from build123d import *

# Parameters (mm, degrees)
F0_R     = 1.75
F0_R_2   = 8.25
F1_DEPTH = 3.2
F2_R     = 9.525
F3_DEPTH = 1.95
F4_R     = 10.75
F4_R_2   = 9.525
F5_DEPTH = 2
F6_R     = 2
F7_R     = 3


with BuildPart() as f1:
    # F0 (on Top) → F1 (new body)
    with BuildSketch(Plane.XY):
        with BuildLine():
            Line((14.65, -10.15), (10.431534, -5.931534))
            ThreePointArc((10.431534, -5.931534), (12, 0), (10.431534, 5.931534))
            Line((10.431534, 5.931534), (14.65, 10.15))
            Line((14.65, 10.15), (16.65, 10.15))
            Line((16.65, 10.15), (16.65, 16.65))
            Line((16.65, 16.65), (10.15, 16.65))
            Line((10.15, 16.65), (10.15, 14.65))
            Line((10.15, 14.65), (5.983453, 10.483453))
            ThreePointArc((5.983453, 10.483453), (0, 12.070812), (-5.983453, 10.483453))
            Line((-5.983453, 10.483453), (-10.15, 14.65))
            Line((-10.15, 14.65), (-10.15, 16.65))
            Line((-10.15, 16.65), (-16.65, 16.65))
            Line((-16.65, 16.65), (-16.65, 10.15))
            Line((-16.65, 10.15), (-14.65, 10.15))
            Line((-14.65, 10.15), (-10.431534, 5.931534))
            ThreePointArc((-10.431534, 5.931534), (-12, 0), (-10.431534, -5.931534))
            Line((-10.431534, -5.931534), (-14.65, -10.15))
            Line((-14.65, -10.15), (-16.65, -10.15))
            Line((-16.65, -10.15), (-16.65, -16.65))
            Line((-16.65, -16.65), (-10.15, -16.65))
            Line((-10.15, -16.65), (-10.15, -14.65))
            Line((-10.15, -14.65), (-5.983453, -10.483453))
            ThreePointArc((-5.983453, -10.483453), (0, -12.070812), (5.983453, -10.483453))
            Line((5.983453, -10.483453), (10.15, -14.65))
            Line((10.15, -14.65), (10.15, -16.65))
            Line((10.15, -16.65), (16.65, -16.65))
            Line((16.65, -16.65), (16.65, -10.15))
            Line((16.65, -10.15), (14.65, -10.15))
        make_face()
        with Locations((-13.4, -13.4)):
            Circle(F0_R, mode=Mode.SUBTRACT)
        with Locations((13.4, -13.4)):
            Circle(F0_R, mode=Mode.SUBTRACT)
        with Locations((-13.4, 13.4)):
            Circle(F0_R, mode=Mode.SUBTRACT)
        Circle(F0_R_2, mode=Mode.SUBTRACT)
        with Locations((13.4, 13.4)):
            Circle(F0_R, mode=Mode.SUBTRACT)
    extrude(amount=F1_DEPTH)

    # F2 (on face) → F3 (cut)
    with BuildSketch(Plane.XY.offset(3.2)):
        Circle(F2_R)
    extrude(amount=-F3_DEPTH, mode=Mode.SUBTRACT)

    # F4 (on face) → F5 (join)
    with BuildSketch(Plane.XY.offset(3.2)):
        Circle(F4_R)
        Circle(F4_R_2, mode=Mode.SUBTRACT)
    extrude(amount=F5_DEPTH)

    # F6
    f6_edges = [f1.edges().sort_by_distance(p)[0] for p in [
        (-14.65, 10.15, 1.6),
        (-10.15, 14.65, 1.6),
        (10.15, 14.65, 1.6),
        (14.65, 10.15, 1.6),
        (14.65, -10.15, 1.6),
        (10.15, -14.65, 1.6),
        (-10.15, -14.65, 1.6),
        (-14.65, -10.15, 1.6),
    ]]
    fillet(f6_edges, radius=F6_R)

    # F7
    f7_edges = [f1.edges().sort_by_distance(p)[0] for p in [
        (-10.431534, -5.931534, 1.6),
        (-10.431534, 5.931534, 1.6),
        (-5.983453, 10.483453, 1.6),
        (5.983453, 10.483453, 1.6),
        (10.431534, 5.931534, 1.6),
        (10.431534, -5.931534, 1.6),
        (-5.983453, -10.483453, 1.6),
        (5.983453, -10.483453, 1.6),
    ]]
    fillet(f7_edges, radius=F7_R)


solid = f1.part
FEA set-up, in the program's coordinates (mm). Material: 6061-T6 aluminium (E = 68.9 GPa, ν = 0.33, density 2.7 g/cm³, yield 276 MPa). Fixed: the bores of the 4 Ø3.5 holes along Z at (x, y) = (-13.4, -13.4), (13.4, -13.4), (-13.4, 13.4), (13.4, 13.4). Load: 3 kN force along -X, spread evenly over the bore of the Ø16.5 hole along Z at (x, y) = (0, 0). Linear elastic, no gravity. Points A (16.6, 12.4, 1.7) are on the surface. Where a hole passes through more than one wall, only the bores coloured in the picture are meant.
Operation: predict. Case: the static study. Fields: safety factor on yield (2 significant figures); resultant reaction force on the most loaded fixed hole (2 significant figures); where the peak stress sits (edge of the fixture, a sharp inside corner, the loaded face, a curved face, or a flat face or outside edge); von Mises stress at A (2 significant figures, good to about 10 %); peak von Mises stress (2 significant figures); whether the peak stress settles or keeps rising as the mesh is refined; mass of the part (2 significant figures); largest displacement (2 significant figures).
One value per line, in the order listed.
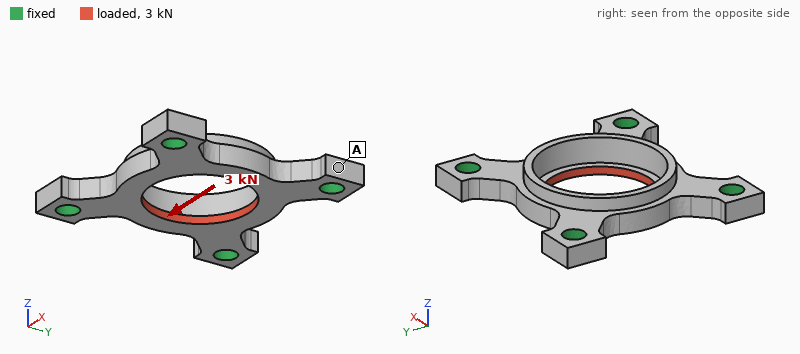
1.4
840 N
the loaded face
29 MPa
190 MPa
settles
4.2 g
37 µm
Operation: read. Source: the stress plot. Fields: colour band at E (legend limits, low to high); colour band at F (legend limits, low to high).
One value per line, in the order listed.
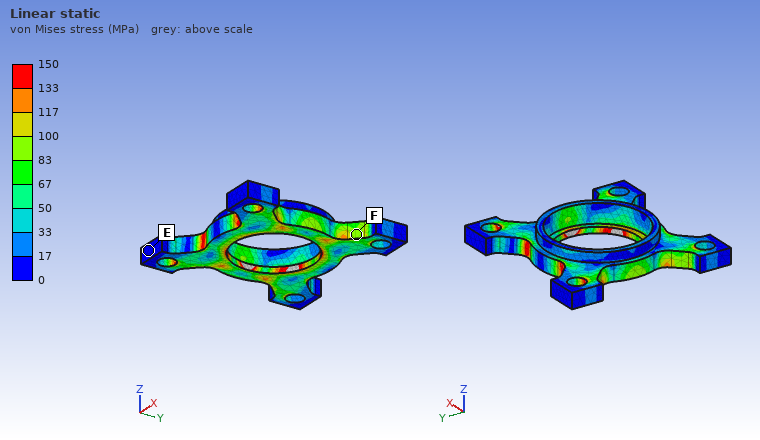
0 to 17 MPa
83 to 100 MPa
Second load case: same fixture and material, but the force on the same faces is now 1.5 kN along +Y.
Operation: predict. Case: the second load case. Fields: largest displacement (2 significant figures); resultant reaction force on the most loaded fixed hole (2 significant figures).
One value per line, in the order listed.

19 µm
420 N
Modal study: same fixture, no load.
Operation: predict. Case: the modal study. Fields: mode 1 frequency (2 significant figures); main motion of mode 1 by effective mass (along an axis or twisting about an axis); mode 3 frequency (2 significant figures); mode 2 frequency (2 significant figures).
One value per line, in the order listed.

22 kHz
along Z
27 kHz
27 kHz
